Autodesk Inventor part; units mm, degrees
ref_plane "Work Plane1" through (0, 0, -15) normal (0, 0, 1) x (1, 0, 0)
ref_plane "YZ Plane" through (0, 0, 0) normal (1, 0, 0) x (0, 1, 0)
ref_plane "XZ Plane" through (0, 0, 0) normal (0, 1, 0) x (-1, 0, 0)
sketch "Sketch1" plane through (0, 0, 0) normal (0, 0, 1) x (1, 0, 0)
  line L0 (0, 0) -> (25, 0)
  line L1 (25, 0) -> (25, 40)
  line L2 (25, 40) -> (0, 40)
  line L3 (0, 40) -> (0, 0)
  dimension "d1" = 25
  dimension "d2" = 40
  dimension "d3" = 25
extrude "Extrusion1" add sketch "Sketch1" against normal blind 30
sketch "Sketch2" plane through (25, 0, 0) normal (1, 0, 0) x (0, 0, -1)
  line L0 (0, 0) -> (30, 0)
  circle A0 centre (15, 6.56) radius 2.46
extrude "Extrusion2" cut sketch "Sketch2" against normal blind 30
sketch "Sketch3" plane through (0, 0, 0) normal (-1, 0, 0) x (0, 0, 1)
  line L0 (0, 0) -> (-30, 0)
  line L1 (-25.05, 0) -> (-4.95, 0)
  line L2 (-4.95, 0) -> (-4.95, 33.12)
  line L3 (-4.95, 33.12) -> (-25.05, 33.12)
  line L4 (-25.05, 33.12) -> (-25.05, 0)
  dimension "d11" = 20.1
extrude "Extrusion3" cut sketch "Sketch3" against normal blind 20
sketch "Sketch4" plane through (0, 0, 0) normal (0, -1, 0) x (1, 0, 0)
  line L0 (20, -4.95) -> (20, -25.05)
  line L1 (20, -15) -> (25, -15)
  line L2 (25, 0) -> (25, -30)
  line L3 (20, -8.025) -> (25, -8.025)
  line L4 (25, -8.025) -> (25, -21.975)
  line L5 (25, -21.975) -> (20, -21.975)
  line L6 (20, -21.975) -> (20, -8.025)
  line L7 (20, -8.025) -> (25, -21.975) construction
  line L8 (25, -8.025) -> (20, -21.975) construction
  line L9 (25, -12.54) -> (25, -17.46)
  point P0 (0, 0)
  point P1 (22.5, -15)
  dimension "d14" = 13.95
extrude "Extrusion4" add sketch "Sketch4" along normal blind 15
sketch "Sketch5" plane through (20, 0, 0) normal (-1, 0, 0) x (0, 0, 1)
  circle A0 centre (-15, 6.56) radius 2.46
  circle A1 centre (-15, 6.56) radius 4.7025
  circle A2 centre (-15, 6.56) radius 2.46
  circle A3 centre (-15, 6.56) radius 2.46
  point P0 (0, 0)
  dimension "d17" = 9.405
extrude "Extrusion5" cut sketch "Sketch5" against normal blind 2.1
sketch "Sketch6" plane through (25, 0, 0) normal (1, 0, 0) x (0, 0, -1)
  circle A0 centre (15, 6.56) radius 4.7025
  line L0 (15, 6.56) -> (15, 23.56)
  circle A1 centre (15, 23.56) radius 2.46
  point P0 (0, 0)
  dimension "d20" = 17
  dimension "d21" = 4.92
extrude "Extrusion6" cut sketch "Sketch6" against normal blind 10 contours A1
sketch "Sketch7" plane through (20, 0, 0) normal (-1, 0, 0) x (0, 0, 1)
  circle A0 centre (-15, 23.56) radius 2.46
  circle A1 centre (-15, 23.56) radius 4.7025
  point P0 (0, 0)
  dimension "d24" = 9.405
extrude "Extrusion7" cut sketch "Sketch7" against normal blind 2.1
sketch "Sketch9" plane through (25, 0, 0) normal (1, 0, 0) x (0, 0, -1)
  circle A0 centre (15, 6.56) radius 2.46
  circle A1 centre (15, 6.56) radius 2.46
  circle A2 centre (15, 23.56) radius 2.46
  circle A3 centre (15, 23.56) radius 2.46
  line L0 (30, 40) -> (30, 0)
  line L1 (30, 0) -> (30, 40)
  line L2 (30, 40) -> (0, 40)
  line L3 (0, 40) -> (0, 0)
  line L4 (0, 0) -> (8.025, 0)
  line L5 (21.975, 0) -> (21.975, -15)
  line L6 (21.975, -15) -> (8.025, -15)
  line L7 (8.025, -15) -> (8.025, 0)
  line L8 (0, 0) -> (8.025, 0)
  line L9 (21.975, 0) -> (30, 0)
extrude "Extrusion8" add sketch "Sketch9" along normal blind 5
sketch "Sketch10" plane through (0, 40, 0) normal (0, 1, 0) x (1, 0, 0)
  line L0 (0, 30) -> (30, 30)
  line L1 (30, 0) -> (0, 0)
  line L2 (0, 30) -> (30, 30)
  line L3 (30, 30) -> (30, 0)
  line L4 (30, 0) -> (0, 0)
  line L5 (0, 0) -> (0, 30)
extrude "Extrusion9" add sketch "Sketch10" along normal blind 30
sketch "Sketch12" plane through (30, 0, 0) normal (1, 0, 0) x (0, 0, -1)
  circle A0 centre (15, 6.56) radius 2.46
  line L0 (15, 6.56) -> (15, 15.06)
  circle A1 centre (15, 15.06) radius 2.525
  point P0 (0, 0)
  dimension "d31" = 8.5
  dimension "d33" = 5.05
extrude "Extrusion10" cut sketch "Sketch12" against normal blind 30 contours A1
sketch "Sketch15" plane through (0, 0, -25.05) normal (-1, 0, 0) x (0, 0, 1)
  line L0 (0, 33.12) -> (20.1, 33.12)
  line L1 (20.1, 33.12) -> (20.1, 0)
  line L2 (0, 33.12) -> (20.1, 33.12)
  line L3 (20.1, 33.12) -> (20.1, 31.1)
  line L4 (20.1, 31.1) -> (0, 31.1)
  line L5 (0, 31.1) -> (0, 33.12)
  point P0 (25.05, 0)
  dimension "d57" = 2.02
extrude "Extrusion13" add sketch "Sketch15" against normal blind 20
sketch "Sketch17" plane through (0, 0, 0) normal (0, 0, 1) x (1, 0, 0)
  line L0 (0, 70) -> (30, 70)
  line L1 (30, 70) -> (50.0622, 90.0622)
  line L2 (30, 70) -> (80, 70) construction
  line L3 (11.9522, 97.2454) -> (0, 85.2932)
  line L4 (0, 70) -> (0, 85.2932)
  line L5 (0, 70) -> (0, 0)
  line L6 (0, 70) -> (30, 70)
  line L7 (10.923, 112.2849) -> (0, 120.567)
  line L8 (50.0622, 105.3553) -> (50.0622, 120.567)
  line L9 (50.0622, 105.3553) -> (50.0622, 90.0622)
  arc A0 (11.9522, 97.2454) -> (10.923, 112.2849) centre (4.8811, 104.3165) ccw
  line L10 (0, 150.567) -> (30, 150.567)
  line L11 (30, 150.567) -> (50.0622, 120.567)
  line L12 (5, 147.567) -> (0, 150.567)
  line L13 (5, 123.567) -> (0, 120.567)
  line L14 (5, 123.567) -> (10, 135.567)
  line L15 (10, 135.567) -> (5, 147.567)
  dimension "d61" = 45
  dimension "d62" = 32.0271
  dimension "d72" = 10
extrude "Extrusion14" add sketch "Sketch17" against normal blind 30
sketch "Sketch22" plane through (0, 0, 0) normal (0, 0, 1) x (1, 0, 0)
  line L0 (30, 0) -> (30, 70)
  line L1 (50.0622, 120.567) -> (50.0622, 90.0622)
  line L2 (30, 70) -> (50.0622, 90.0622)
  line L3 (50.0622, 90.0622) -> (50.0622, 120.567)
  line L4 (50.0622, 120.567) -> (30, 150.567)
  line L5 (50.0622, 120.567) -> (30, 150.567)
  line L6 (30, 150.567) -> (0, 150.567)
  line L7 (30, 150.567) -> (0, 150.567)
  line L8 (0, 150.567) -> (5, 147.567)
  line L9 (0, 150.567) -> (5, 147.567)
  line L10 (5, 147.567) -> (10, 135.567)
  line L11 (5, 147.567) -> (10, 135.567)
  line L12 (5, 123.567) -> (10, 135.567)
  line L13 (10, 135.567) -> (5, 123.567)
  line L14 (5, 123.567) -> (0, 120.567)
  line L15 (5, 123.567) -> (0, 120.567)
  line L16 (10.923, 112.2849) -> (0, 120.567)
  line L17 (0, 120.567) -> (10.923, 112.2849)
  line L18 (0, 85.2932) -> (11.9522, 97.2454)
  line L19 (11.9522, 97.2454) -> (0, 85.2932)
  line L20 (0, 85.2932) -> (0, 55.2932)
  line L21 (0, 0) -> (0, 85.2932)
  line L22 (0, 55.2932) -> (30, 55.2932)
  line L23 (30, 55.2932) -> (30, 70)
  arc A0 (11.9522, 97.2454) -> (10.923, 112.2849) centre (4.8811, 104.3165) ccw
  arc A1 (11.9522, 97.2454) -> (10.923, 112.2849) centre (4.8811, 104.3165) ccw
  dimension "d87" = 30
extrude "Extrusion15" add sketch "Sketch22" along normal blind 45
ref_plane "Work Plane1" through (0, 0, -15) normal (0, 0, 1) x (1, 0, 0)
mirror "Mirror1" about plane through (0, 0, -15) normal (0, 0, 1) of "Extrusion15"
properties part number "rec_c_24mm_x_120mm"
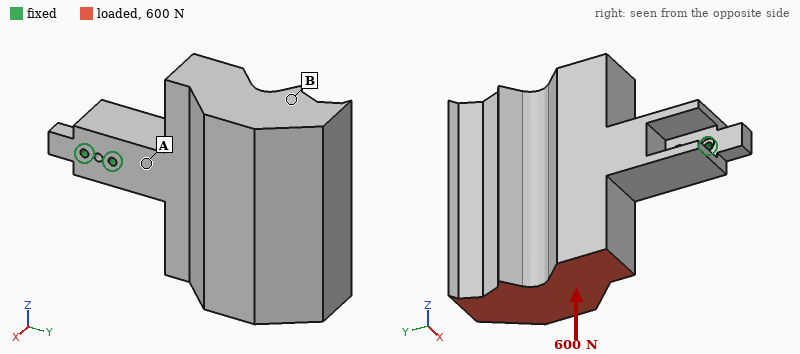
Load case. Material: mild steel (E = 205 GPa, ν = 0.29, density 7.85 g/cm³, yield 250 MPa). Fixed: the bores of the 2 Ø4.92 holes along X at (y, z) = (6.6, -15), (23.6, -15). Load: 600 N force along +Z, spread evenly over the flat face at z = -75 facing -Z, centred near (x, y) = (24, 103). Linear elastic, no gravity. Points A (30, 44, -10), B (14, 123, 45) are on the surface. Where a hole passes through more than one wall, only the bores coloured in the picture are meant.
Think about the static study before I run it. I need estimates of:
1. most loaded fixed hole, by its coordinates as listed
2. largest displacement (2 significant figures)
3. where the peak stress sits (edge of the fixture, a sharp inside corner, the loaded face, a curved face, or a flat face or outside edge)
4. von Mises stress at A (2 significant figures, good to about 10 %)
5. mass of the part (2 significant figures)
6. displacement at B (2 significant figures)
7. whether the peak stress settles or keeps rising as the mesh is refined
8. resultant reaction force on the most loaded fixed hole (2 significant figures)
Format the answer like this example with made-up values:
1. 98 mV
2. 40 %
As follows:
1. (23.6, -15)
2. 46 µm
3. edge of the fixture
4. 6.8 MPa
5. 3.6 kg
6. 37 µm
7. keeps rising
8. 2.6 kN
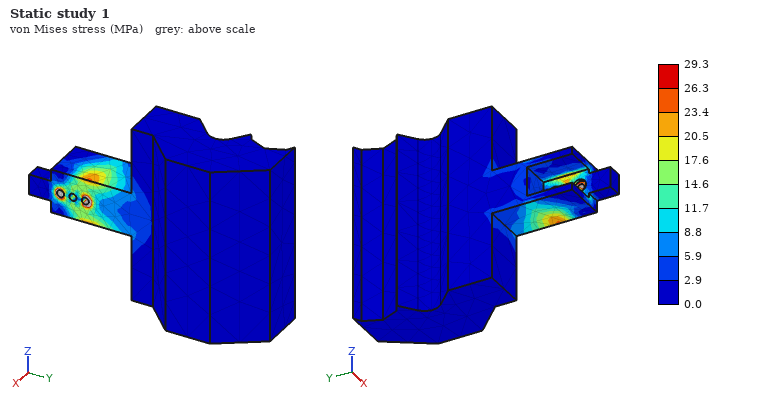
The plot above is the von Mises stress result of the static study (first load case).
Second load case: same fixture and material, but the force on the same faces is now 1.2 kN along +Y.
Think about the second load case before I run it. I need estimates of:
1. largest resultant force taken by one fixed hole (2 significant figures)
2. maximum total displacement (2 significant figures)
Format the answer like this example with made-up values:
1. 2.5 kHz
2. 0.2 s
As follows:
1. 3.2 kN
2. 77 µm
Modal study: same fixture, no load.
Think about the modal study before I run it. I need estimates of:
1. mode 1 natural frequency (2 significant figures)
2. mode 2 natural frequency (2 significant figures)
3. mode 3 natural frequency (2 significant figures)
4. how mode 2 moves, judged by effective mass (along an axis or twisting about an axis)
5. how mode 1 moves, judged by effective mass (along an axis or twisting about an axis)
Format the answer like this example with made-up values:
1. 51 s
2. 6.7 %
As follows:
1. 350 Hz
2. 370 Hz
3. 560 Hz
4. along Z
5. along X
